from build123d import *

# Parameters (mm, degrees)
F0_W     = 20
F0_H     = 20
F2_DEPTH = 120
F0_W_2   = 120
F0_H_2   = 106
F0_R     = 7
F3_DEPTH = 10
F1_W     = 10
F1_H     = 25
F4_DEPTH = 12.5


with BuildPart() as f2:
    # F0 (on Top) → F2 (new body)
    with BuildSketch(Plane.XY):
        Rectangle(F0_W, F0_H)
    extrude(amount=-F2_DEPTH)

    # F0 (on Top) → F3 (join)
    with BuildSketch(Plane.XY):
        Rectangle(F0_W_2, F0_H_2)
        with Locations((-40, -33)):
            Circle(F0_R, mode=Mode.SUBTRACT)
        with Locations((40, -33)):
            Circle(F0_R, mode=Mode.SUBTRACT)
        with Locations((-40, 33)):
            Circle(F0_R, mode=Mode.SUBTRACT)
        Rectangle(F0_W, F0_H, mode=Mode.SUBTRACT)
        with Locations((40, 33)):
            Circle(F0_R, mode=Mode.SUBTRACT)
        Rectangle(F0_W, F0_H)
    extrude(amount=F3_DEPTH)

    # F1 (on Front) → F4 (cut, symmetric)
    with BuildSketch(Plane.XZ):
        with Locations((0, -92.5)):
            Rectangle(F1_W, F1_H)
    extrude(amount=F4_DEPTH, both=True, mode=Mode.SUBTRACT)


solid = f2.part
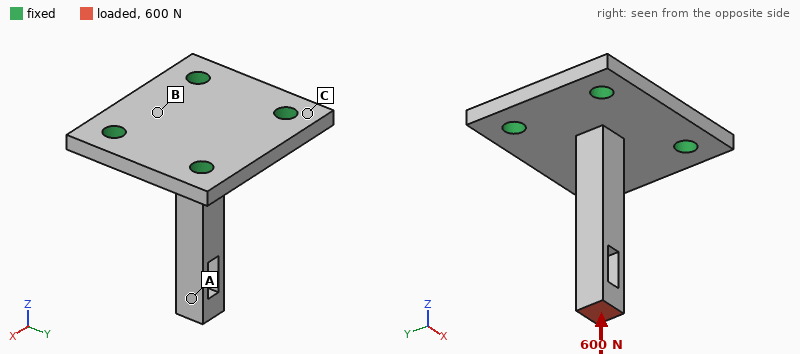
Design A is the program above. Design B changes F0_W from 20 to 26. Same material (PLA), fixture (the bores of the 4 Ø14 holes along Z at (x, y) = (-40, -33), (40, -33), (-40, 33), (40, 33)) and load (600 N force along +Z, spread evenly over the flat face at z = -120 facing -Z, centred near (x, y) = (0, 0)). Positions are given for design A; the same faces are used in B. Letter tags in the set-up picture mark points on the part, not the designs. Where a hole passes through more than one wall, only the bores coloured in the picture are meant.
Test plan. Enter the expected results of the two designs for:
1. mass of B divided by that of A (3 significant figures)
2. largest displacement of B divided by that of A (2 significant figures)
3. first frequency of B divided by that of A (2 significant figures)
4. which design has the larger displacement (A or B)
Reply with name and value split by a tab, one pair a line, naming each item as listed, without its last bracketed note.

mass of B divided by that of A	1.09
largest displacement of B divided by that of A	0.81
first frequency of B divided by that of A	0.96
which design has the larger displacement	A
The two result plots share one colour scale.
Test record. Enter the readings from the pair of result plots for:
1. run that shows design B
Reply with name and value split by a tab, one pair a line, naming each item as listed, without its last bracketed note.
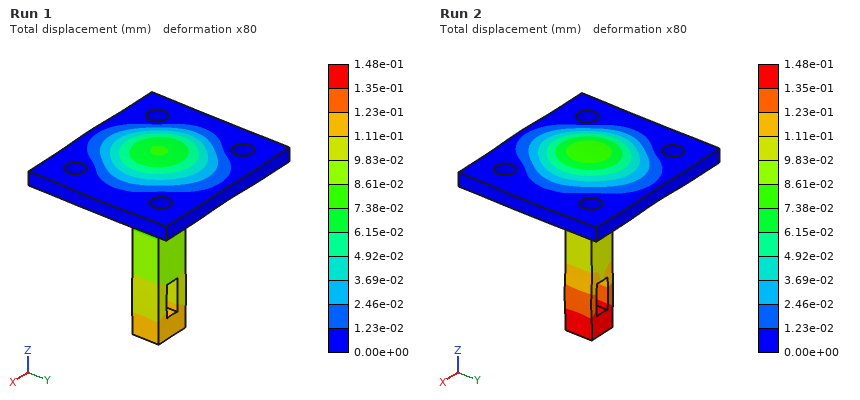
run that shows design B	Run 1
